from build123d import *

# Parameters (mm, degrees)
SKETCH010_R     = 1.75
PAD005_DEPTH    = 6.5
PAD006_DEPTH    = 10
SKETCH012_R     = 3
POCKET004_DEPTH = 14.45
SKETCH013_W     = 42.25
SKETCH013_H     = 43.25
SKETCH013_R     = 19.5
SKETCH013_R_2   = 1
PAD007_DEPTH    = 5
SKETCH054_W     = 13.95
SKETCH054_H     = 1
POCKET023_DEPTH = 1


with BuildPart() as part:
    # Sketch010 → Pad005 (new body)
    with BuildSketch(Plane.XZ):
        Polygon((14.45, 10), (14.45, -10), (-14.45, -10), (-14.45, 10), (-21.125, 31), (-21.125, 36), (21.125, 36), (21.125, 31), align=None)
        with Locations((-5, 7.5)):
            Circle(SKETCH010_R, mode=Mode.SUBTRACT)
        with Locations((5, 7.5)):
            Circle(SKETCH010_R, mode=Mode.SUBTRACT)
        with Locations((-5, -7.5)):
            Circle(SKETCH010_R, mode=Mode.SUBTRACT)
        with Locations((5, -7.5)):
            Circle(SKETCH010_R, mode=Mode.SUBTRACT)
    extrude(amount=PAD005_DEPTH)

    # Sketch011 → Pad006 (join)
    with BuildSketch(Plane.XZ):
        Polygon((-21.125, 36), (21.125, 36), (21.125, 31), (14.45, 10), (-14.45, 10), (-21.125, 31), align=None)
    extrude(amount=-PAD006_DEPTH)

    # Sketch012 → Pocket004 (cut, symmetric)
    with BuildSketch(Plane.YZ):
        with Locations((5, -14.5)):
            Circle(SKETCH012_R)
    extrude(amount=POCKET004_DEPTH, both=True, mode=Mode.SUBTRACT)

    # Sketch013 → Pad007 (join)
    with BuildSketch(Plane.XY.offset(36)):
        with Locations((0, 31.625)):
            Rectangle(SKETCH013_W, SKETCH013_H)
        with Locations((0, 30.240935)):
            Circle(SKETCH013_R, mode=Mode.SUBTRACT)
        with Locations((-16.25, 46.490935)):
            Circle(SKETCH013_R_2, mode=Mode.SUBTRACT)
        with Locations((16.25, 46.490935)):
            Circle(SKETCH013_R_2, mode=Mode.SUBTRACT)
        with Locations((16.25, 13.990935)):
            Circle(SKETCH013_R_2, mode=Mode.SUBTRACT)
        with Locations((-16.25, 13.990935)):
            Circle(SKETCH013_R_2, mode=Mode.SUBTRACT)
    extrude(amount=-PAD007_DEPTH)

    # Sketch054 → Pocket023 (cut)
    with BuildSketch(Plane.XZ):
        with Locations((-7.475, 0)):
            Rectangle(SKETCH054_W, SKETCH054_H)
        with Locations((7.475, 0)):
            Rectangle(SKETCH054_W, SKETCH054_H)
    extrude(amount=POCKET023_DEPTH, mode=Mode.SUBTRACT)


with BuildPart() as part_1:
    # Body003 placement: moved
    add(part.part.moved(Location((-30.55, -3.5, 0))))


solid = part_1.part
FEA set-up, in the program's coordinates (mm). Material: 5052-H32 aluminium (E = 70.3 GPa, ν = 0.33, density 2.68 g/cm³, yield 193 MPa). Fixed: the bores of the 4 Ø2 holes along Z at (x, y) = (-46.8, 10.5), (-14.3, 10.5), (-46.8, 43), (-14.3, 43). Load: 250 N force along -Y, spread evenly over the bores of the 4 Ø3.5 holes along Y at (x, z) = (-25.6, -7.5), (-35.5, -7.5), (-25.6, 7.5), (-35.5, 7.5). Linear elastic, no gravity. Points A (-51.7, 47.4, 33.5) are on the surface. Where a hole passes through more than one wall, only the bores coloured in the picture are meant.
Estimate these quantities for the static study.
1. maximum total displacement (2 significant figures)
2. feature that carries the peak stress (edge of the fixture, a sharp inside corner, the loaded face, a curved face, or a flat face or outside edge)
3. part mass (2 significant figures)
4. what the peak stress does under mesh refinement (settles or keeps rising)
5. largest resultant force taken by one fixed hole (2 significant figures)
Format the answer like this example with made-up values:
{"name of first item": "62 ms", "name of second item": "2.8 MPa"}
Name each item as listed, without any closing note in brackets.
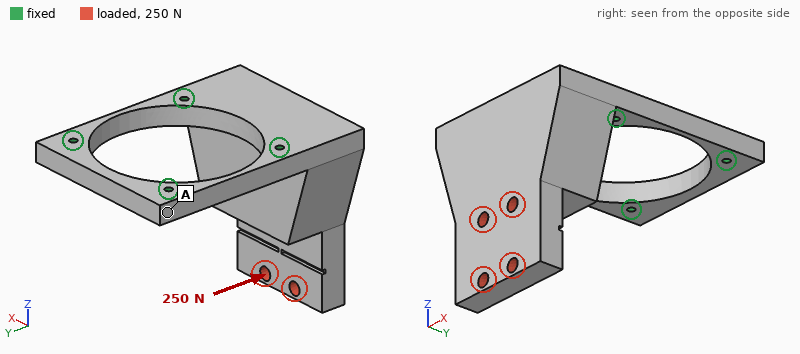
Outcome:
{"maximum total displacement": "0.20 mm", "feature that carries the peak stress": "edge of the fixture", "part mass": "60 g", "what the peak stress does under mesh refinement": "keeps rising", "largest resultant force taken by one fixed hole": "130 N"}
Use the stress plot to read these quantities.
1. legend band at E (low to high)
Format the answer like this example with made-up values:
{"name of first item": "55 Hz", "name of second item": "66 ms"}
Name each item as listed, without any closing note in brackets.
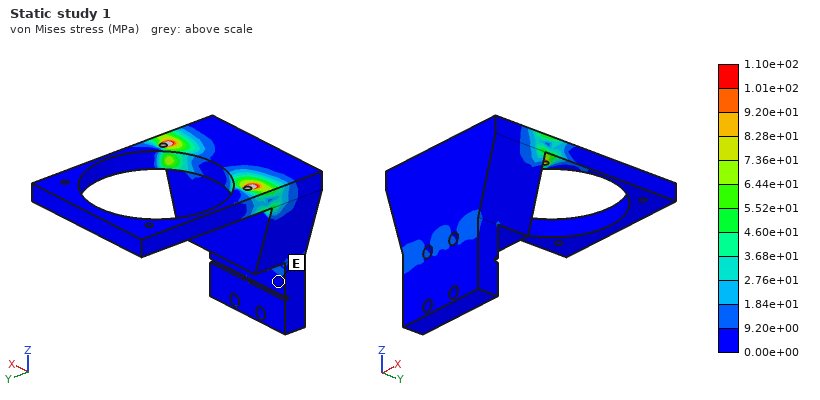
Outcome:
{"legend band at E": "0.00e+00 to 9.20e+00 MPa"}
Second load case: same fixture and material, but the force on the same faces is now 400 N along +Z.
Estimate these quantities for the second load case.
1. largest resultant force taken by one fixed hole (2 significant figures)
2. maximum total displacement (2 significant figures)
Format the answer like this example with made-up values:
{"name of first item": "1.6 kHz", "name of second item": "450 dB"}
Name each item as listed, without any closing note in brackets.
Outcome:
{"largest resultant force taken by one fixed hole": "210 N", "maximum total displacement": "0.13 mm"}
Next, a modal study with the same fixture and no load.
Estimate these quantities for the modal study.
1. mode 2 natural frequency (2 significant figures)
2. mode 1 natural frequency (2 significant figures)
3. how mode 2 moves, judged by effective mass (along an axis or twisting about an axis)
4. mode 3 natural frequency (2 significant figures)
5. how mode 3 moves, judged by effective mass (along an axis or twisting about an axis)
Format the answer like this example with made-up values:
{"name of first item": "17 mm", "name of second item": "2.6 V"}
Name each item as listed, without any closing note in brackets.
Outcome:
{"mode 2 natural frequency": "6600 Hz", "mode 1 natural frequency": "1500 Hz", "how mode 2 moves, judged by effective mass": "along X", "mode 3 natural frequency": "9300 Hz", "how mode 3 moves, judged by effective mass": "along Z"}
